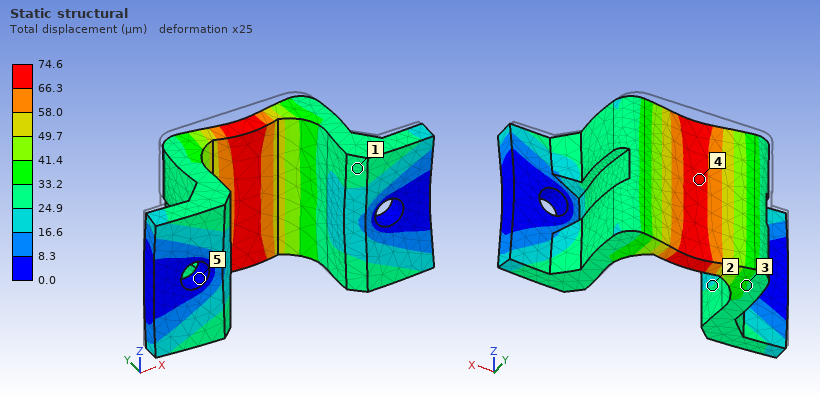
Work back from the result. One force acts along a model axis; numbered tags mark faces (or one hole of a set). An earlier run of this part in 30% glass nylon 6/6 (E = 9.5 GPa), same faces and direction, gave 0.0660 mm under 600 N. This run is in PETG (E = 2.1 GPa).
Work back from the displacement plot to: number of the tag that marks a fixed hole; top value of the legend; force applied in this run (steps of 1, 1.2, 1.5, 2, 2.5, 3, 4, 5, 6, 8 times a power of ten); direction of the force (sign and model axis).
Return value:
5
74.6 µm
150 N
-Y
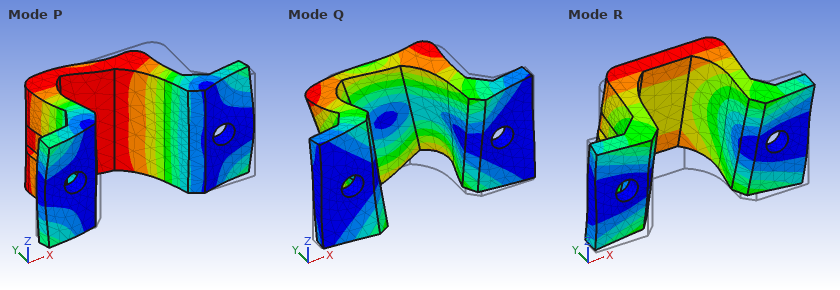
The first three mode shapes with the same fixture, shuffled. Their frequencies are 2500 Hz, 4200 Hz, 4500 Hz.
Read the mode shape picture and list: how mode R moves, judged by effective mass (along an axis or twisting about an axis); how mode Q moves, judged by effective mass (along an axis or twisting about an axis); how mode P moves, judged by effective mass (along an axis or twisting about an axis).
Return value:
along Z
twisting about Y
along X
